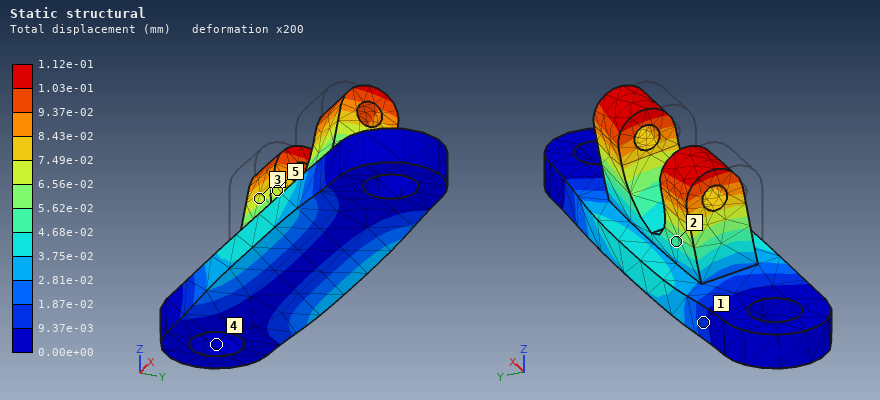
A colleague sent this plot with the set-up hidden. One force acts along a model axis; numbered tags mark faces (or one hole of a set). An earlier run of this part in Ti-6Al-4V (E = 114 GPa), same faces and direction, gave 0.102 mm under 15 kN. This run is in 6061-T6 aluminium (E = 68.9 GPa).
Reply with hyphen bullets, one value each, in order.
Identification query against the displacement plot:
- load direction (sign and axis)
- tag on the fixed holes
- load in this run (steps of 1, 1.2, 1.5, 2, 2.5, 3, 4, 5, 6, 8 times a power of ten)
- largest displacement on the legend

- +Y
- 4
- 10 kN
- 1.12e-01 mm
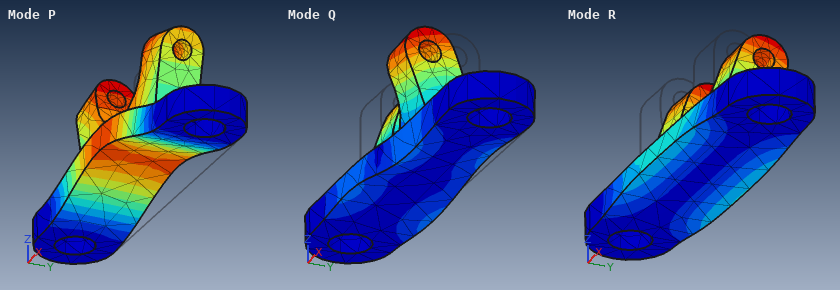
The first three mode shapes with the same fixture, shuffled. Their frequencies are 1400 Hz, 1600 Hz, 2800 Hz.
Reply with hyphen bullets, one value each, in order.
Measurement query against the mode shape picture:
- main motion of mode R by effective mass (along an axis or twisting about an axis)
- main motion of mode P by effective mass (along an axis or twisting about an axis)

- along Y
- along Z
